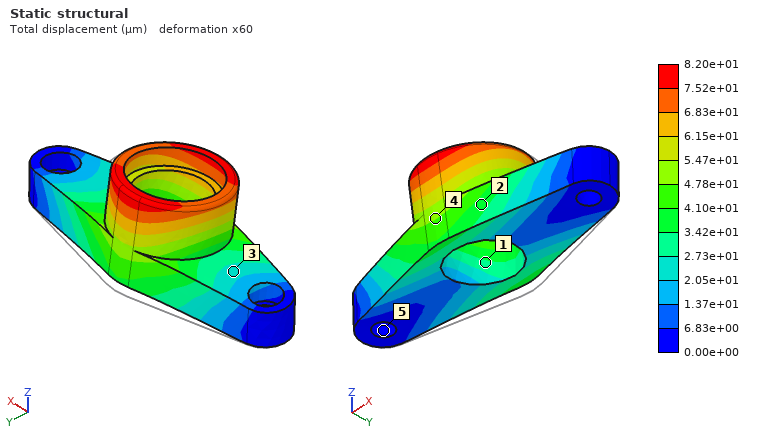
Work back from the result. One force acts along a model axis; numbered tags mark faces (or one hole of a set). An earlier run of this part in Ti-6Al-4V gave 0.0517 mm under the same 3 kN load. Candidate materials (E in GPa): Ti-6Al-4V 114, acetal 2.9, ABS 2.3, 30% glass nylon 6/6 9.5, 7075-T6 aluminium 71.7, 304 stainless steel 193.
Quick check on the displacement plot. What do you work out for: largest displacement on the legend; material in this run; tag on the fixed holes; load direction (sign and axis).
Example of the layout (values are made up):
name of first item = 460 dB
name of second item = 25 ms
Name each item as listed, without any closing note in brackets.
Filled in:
largest displacement on the legend = 8.20e+01 µm
material in this run = 7075-T6 aluminium
tag on the fixed holes = 5
load direction = -Y
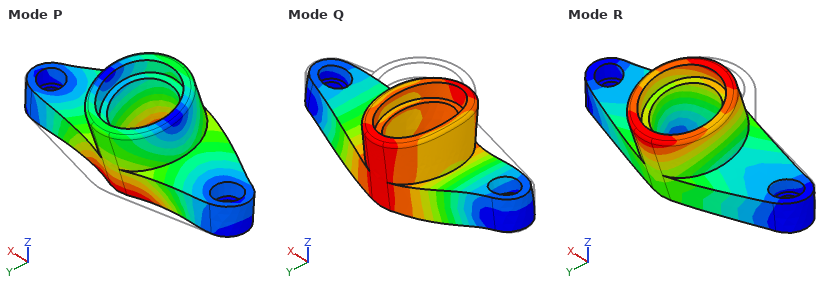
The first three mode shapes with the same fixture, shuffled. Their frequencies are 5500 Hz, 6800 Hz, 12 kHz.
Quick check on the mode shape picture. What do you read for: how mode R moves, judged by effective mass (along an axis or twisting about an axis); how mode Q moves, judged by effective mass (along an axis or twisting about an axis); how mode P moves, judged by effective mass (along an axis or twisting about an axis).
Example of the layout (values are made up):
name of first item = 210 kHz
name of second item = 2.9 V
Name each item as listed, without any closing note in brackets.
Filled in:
how mode R moves, judged by effective mass = along Y
how mode Q moves, judged by effective mass = along Z
how mode P moves, judged by effective mass = along Y
